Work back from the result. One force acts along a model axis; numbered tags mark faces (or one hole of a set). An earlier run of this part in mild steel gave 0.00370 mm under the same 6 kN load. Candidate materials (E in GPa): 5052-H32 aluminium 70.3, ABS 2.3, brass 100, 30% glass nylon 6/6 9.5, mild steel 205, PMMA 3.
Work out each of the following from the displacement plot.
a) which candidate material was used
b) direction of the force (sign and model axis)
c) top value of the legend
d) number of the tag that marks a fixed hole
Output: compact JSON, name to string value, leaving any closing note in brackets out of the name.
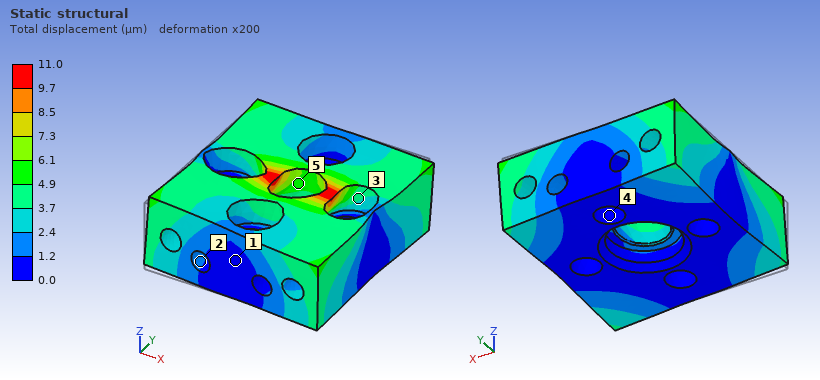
{"which candidate material was used": "5052-H32 aluminium", "direction of the force": "+X", "top value of the legend": "11.0 µm", "number of the tag that marks a fixed hole": "4"}
